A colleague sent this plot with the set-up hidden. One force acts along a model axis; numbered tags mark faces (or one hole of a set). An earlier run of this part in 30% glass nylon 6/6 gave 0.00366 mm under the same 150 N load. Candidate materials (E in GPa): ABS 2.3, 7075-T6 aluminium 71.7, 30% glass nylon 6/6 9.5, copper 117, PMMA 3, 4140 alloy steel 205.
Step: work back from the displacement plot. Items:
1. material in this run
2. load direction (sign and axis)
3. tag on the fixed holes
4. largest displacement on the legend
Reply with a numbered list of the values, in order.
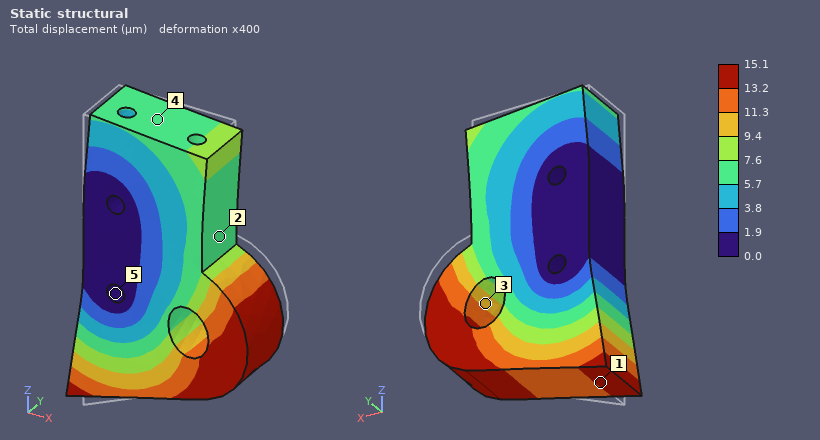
1. ABS
2. -Z
3. 5
4. 15.1 µm
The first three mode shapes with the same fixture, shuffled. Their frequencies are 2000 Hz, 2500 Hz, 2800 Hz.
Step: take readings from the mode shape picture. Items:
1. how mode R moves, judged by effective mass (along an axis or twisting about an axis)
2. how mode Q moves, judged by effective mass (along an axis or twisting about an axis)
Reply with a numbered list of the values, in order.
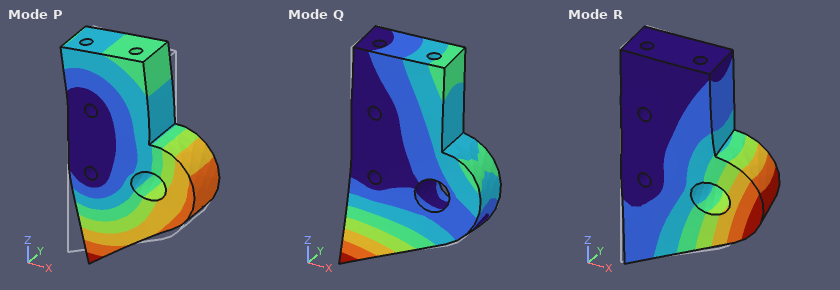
1. along Y
2. twisting about X
